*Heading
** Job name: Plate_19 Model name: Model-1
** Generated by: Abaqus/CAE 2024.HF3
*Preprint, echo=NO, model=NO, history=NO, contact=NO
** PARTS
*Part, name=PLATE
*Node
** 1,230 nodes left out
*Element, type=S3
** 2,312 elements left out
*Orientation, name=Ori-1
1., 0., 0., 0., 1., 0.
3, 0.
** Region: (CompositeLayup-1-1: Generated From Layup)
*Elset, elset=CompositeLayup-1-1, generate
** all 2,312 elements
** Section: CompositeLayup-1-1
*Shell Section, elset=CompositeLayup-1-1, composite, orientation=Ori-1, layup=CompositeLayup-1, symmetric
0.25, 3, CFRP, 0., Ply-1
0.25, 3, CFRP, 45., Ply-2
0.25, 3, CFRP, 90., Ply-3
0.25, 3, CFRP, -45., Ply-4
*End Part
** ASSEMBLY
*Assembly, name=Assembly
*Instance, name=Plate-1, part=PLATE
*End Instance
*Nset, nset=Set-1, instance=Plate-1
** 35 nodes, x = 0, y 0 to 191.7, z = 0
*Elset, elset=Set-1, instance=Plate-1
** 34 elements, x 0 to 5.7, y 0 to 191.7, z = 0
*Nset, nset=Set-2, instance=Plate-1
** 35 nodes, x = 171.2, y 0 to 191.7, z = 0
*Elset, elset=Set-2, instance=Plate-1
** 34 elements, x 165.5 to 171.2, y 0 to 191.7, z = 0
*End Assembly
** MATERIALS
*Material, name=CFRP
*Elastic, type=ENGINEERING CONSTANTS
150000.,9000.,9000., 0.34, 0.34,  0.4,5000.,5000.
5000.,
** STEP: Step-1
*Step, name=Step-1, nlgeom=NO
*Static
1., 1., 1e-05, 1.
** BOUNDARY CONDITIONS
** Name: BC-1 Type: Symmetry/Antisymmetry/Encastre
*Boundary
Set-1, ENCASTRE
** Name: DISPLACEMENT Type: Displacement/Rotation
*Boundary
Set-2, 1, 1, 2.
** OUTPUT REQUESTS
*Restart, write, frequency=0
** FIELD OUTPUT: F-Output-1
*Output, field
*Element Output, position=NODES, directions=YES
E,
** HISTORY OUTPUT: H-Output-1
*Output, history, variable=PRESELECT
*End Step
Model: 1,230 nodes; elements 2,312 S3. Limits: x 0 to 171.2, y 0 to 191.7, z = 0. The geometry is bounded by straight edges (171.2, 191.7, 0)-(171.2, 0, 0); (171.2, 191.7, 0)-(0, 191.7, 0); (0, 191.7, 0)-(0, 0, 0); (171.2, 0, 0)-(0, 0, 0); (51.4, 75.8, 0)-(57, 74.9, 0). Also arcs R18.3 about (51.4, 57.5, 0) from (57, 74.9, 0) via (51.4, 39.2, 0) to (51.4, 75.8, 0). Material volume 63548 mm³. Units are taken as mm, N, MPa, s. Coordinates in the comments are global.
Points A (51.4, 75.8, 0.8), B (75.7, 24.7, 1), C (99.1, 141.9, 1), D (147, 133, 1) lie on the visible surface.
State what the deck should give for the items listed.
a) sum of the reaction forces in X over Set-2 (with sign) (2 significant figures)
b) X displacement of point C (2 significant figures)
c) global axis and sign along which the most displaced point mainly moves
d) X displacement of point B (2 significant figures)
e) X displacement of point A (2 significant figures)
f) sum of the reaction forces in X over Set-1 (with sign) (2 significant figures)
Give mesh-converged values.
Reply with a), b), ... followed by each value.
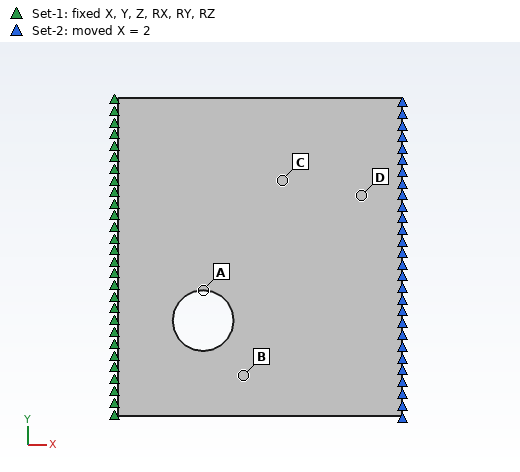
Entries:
a) 2.4e+05 N
b) 1.1 mm
c) +X
d) 0.98 mm
e) 0.63 mm
f) -2.4e+05 N
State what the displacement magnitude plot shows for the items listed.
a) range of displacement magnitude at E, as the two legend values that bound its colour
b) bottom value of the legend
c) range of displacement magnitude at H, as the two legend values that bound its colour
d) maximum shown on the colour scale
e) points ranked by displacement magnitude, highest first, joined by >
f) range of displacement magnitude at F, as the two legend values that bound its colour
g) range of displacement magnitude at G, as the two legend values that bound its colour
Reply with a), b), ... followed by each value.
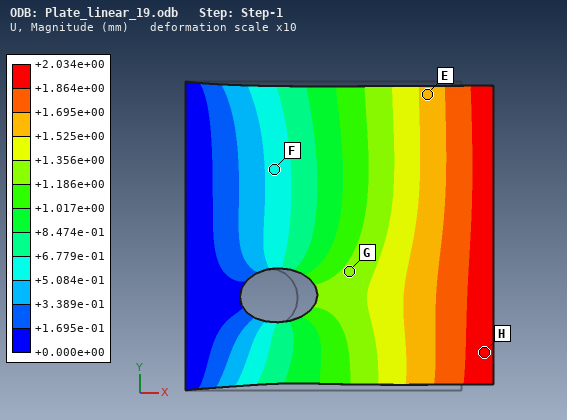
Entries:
a) +1.525e+00 to +1.695e+00 mm
b) +0.000e+00 mm
c) +1.864e+00 to +2.034e+00 mm
d) +2.034e+00 mm
e) H > E > G > F
f) +5.084e-01 to +6.779e-01 mm
g) +1.186e+00 to +1.356e+00 mm
